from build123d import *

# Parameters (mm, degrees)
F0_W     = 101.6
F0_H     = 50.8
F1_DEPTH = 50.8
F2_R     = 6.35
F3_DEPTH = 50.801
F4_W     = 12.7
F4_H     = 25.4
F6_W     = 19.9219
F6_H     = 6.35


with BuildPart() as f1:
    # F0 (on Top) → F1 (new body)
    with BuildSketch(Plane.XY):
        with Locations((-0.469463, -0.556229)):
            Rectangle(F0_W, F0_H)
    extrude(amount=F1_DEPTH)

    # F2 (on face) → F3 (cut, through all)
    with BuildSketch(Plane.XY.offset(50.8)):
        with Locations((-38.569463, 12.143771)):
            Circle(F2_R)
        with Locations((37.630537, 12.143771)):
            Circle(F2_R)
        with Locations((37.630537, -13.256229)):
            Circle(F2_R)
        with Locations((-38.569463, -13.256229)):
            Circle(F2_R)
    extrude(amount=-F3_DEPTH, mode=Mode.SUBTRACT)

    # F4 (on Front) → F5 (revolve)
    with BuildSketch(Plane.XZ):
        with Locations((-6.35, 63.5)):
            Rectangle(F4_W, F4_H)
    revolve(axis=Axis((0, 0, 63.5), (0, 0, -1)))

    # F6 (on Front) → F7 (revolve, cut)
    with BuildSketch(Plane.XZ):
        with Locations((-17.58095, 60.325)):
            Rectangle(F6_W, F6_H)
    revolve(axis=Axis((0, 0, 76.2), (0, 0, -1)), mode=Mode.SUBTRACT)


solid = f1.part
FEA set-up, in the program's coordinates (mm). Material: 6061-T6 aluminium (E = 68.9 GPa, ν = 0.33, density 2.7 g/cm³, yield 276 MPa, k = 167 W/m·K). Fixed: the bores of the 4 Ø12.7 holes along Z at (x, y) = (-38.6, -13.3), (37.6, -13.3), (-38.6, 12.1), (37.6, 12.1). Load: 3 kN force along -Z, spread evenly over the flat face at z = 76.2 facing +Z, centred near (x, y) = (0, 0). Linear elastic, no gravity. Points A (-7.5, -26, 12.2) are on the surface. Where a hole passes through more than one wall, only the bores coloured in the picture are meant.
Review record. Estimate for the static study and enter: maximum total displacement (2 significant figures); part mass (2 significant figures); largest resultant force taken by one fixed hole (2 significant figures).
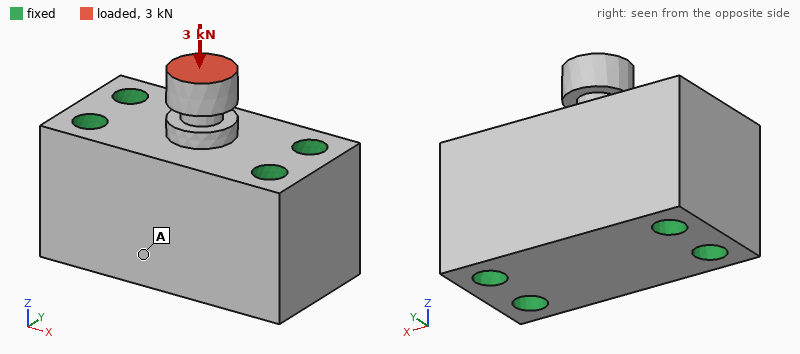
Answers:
6.0 µm
670 g
810 N
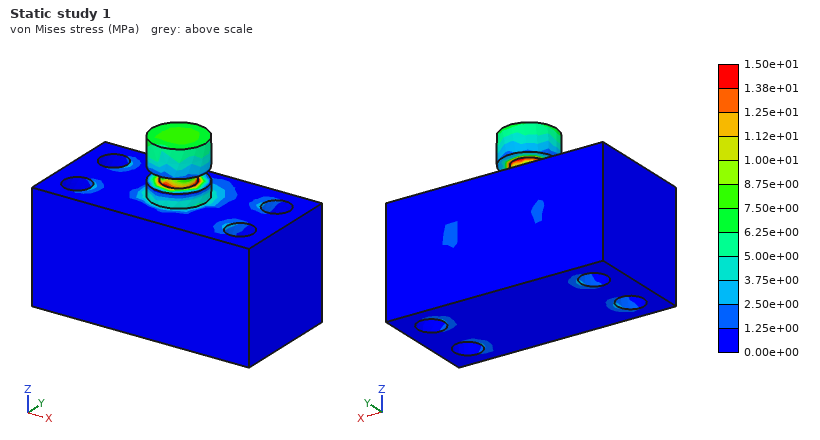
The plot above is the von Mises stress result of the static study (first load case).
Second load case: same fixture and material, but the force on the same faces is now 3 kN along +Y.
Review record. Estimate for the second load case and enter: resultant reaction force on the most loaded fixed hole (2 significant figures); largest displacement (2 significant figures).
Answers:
1.8 kN
89 µm
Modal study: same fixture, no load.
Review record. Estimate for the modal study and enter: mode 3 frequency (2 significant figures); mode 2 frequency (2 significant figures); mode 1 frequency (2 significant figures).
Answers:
15 kHz
9900 Hz
9500 Hz
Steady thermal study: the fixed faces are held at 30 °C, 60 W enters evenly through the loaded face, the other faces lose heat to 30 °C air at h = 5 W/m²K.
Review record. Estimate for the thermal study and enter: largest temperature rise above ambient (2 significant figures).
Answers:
39 K
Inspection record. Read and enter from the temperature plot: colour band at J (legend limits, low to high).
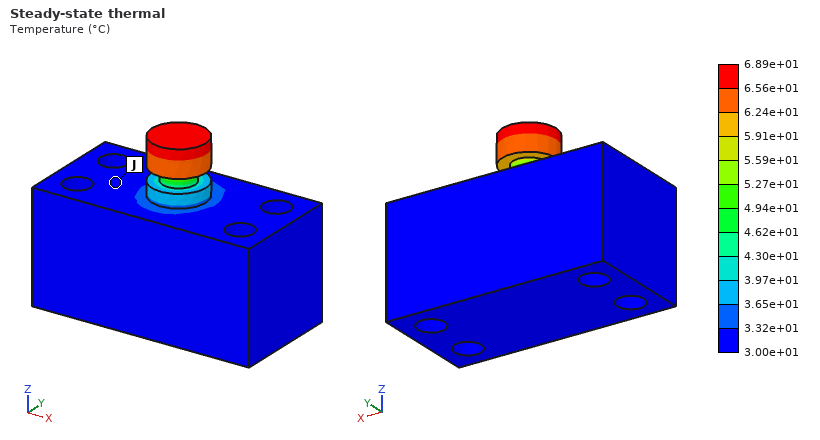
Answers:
3.00e+01 to 3.32e+01 °C
